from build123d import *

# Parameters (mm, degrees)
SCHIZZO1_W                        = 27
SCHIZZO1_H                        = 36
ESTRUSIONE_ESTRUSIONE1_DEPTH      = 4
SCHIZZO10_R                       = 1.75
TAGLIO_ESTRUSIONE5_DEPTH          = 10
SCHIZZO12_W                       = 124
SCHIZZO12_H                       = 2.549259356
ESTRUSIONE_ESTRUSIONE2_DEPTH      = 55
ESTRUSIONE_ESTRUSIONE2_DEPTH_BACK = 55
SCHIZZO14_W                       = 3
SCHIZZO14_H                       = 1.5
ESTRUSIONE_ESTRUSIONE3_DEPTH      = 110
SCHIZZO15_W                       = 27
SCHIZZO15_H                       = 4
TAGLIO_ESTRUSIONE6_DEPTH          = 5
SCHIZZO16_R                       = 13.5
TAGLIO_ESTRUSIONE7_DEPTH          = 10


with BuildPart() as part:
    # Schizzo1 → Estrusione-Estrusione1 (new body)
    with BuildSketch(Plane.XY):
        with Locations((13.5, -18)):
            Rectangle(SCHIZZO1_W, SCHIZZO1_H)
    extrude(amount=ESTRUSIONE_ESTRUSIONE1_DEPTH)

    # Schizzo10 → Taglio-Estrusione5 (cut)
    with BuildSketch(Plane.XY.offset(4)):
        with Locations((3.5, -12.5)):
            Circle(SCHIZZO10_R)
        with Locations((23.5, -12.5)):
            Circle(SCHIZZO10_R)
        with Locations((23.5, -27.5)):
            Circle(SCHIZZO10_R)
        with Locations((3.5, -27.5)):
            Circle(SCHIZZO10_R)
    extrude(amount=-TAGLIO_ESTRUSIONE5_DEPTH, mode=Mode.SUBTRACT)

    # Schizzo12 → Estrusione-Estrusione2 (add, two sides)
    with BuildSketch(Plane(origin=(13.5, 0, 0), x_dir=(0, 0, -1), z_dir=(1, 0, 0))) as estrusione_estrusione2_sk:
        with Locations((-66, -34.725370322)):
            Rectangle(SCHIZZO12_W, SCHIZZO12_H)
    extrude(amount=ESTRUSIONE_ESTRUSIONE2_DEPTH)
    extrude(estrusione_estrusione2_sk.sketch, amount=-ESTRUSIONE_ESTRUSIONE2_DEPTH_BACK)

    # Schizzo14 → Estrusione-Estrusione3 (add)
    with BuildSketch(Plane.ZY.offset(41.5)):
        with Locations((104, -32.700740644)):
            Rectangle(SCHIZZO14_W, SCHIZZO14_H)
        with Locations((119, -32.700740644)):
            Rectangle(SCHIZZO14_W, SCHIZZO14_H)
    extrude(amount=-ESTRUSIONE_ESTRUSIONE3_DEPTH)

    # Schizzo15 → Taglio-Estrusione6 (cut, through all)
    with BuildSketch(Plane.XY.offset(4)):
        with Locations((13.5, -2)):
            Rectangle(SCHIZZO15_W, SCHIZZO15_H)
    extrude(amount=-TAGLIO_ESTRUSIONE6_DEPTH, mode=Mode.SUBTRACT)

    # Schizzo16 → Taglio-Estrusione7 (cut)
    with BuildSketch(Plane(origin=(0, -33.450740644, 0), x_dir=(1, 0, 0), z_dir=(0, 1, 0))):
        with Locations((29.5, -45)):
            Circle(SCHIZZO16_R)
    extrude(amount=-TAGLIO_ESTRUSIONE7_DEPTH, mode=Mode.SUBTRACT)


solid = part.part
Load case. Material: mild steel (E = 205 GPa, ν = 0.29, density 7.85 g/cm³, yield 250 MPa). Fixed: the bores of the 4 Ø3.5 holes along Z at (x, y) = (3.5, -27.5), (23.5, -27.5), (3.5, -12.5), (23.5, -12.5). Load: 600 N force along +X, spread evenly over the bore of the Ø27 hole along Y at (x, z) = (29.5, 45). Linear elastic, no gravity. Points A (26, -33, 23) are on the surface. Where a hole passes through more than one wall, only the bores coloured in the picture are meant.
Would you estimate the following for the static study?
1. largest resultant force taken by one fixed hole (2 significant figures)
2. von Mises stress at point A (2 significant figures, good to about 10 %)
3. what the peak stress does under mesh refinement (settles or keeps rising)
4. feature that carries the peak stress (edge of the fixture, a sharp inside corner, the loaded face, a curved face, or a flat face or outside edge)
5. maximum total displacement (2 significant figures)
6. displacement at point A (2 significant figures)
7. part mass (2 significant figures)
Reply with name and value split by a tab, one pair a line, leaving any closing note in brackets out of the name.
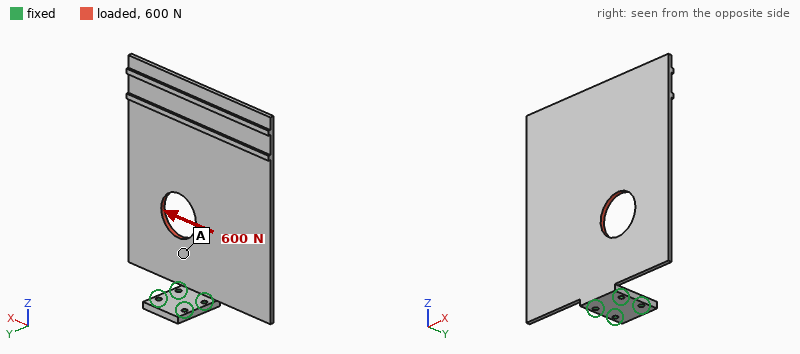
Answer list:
largest resultant force taken by one fixed hole	1.3 kN
von Mises stress at point A	21 MPa
what the peak stress does under mesh refinement	keeps rising
feature that carries the peak stress	edge of the fixture
maximum total displacement	0.19 mm
displacement at point A	0.035 mm
part mass	300 g
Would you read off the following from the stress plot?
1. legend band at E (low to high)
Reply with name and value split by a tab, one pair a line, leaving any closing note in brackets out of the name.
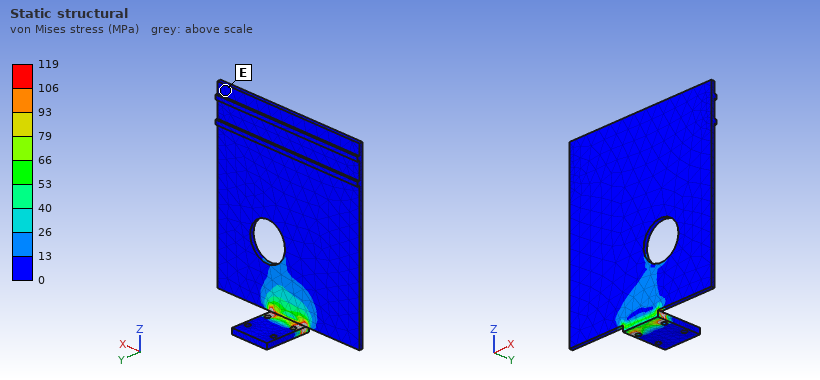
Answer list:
legend band at E	0 to 13 MPa
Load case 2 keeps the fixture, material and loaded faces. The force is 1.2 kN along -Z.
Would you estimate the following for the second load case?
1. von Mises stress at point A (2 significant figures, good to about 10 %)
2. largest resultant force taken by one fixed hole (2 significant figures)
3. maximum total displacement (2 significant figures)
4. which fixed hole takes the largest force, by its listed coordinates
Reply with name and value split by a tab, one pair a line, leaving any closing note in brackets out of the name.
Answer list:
von Mises stress at point A	18 MPa
largest resultant force taken by one fixed hole	1.6 kN
maximum total displacement	0.23 mm
which fixed hole takes the largest force, by its listed coordinates	(23.5, -27.5)
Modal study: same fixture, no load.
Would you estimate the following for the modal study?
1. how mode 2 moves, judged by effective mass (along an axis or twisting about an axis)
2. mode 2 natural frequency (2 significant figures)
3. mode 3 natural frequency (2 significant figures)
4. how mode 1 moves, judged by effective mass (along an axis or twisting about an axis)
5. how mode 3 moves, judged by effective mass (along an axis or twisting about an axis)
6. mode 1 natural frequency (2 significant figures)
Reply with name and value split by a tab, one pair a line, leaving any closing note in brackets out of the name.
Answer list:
how mode 2 moves, judged by effective mass	twisting about Z
mode 2 natural frequency	230 Hz
mode 3 natural frequency	530 Hz
how mode 1 moves, judged by effective mass	along Y
how mode 3 moves, judged by effective mass	along X
mode 1 natural frequency	91 Hz
